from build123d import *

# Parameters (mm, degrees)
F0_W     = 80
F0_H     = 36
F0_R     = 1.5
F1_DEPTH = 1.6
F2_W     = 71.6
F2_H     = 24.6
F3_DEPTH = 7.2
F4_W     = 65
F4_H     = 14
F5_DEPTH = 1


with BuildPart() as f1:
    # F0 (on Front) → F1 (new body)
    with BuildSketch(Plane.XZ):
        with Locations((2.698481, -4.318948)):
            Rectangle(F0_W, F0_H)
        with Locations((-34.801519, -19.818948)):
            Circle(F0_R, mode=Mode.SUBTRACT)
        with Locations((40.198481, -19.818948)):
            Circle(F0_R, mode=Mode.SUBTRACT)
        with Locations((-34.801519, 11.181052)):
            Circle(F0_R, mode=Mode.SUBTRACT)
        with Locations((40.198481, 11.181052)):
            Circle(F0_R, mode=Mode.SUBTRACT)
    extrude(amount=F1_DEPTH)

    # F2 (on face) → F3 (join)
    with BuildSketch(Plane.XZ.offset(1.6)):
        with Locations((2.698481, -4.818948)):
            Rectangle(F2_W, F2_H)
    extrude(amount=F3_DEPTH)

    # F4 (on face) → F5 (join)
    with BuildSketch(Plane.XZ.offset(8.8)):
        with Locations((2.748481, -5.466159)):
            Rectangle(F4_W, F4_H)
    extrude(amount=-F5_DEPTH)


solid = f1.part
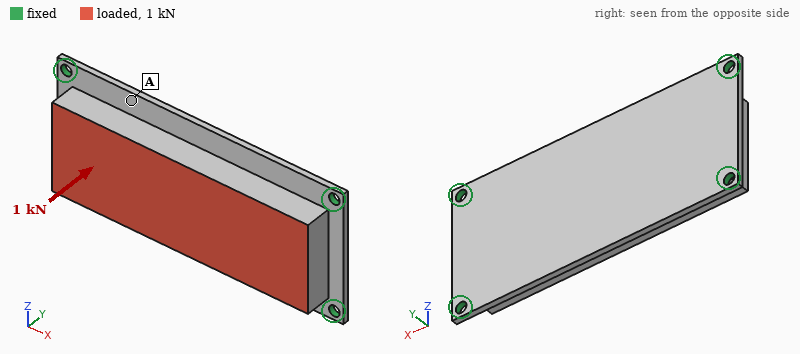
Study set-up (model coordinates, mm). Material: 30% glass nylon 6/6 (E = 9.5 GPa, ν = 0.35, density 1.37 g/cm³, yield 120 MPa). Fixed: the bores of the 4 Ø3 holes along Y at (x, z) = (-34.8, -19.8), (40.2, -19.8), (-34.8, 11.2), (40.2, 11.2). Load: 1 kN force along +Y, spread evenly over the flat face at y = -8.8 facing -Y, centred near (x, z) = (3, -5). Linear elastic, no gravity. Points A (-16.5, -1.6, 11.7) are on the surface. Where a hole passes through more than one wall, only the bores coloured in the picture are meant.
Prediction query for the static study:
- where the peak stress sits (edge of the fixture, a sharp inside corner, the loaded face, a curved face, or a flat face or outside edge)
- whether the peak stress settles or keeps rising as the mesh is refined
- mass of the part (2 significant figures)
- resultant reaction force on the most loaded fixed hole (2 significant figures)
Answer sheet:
edge of the fixture
keeps rising
24 g
470 N
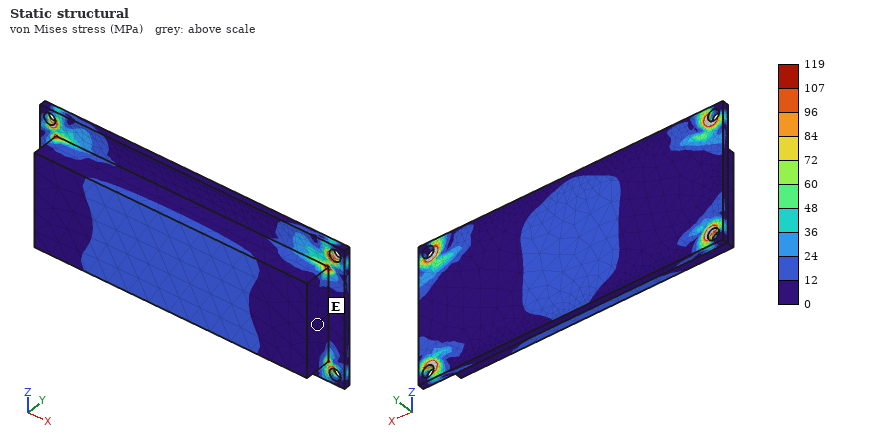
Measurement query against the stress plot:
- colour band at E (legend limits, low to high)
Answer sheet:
0 to 12 MPa
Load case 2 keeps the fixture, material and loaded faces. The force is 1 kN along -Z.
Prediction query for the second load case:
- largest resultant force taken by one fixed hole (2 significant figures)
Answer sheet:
350 N
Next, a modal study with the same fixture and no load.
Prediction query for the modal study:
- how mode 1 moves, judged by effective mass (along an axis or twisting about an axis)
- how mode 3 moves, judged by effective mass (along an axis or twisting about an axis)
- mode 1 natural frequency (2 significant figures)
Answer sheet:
along Y
twisting about Z
2000 Hz
